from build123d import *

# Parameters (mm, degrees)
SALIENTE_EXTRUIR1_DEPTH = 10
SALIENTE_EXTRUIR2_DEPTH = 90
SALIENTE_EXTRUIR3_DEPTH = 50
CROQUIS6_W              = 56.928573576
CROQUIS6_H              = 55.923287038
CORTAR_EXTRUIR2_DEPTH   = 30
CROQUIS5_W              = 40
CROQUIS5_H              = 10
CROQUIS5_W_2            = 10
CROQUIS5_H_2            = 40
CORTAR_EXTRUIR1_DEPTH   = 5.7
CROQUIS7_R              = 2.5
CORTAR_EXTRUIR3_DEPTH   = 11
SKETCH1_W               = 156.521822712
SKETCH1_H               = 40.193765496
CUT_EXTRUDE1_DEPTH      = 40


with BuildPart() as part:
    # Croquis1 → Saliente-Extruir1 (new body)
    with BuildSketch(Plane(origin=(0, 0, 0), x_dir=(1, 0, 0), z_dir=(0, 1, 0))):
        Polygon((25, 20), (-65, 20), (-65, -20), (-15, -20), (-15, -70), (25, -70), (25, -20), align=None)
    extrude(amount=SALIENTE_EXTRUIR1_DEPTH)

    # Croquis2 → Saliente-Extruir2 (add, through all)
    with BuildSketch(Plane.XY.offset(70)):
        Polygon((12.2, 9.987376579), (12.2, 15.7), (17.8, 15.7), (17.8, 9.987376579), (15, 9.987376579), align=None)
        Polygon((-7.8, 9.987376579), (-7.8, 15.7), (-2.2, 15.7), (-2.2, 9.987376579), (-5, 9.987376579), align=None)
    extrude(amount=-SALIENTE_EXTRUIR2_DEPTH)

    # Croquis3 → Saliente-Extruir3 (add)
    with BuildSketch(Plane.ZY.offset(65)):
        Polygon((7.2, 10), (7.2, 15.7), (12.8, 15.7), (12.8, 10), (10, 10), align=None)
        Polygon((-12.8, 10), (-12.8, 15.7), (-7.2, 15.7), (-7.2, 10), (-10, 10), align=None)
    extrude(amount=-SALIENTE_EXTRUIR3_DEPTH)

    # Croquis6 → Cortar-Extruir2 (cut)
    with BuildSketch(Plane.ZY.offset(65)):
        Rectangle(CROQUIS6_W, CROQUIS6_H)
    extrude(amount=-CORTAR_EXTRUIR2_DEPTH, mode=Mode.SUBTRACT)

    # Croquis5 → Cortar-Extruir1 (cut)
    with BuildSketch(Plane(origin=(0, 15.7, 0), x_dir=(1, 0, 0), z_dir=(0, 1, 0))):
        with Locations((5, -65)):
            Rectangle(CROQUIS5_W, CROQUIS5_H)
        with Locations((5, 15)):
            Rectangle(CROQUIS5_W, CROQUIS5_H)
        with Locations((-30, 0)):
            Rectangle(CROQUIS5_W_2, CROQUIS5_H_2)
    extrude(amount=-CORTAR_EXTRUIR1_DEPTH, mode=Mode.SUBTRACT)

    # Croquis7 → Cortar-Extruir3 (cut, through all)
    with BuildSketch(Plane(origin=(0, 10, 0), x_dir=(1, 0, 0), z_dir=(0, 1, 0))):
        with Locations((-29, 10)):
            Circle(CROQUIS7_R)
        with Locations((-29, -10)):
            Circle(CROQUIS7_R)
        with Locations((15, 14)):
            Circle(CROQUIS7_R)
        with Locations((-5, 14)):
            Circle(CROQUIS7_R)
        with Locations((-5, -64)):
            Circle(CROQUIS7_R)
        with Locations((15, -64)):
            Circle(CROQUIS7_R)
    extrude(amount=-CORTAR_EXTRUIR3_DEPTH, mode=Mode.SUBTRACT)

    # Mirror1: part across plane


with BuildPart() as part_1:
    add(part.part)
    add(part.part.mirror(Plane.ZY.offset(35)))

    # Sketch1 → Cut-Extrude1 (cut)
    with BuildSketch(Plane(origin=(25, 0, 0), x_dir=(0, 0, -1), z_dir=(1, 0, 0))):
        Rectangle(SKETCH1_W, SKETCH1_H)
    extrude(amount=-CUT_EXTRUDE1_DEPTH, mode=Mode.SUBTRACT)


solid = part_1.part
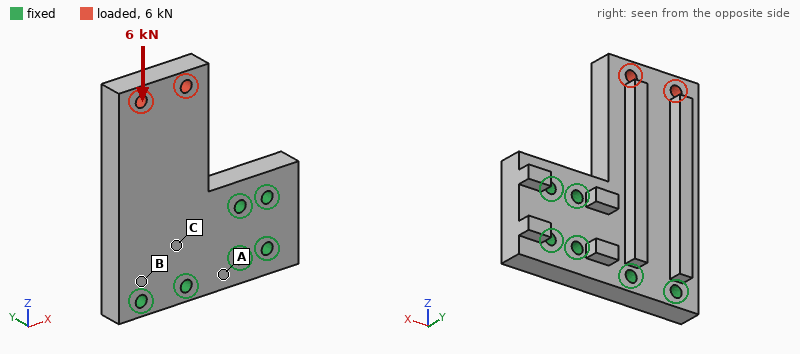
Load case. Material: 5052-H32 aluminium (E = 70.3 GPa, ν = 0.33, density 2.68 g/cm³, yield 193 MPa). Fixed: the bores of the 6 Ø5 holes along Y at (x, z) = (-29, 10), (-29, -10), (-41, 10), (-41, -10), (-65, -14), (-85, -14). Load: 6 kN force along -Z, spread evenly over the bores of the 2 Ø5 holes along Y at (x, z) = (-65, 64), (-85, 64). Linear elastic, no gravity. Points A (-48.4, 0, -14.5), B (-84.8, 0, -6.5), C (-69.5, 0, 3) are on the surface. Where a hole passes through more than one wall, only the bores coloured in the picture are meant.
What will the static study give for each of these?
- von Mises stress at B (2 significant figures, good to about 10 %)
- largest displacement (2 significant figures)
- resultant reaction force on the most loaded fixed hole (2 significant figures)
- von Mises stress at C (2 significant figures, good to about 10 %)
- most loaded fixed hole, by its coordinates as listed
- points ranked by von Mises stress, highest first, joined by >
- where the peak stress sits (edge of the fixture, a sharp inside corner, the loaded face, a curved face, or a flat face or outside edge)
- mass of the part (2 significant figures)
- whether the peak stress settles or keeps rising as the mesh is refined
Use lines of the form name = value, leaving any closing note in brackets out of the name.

von Mises stress at B = 23 MPa
largest displacement = 39 µm
resultant reaction force on the most loaded fixed hole = 3.2 kN
von Mises stress at C = 15 MPa
most loaded fixed hole, by its coordinates as listed = (-85, -14)
points ranked by von Mises stress, highest first, joined by > = B > C > A
where the peak stress sits = edge of the fixture
mass of the part = 150 g
whether the peak stress settles or keeps rising as the mesh is refined = keeps rising
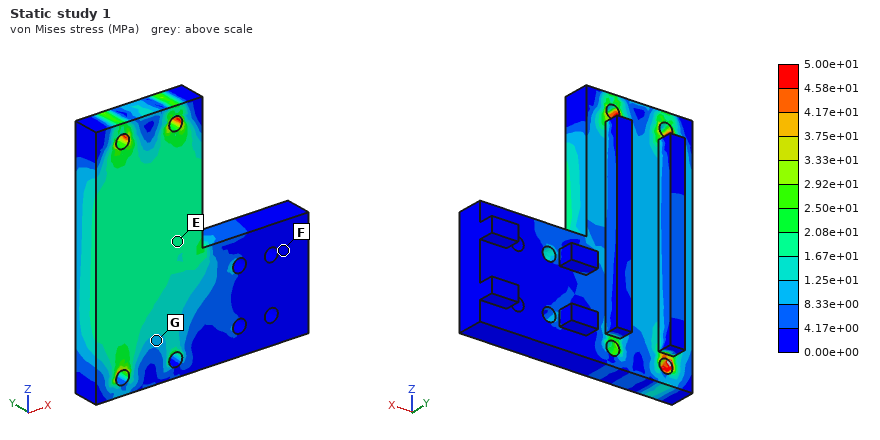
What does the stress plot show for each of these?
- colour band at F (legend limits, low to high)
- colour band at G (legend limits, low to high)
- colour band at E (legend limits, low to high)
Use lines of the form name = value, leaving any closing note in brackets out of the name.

colour band at F = 0.00e+00 to 4.17e+00 MPa
colour band at G = 8.33e+00 to 1.25e+01 MPa
colour band at E = 1.67e+01 to 2.08e+01 MPa
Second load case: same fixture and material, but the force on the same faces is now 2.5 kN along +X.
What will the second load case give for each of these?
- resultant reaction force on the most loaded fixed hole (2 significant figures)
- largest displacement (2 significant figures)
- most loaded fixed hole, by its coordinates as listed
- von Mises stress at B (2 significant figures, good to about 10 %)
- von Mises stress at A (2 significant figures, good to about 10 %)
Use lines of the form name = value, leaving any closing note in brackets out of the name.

resultant reaction force on the most loaded fixed hole = 3.4 kN
largest displacement = 78 µm
most loaded fixed hole, by its coordinates as listed = (-85, -14)
von Mises stress at B = 24 MPa
von Mises stress at A = 4.4 MPa
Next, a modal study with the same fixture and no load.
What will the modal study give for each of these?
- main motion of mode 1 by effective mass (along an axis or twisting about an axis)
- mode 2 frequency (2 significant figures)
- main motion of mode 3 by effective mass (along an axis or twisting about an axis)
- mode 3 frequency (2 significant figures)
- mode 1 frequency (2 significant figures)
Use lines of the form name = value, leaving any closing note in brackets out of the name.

main motion of mode 1 by effective mass = along Y
mode 2 frequency = 5700 Hz
main motion of mode 3 by effective mass = along X
mode 3 frequency = 5900 Hz
mode 1 frequency = 1800 Hz
